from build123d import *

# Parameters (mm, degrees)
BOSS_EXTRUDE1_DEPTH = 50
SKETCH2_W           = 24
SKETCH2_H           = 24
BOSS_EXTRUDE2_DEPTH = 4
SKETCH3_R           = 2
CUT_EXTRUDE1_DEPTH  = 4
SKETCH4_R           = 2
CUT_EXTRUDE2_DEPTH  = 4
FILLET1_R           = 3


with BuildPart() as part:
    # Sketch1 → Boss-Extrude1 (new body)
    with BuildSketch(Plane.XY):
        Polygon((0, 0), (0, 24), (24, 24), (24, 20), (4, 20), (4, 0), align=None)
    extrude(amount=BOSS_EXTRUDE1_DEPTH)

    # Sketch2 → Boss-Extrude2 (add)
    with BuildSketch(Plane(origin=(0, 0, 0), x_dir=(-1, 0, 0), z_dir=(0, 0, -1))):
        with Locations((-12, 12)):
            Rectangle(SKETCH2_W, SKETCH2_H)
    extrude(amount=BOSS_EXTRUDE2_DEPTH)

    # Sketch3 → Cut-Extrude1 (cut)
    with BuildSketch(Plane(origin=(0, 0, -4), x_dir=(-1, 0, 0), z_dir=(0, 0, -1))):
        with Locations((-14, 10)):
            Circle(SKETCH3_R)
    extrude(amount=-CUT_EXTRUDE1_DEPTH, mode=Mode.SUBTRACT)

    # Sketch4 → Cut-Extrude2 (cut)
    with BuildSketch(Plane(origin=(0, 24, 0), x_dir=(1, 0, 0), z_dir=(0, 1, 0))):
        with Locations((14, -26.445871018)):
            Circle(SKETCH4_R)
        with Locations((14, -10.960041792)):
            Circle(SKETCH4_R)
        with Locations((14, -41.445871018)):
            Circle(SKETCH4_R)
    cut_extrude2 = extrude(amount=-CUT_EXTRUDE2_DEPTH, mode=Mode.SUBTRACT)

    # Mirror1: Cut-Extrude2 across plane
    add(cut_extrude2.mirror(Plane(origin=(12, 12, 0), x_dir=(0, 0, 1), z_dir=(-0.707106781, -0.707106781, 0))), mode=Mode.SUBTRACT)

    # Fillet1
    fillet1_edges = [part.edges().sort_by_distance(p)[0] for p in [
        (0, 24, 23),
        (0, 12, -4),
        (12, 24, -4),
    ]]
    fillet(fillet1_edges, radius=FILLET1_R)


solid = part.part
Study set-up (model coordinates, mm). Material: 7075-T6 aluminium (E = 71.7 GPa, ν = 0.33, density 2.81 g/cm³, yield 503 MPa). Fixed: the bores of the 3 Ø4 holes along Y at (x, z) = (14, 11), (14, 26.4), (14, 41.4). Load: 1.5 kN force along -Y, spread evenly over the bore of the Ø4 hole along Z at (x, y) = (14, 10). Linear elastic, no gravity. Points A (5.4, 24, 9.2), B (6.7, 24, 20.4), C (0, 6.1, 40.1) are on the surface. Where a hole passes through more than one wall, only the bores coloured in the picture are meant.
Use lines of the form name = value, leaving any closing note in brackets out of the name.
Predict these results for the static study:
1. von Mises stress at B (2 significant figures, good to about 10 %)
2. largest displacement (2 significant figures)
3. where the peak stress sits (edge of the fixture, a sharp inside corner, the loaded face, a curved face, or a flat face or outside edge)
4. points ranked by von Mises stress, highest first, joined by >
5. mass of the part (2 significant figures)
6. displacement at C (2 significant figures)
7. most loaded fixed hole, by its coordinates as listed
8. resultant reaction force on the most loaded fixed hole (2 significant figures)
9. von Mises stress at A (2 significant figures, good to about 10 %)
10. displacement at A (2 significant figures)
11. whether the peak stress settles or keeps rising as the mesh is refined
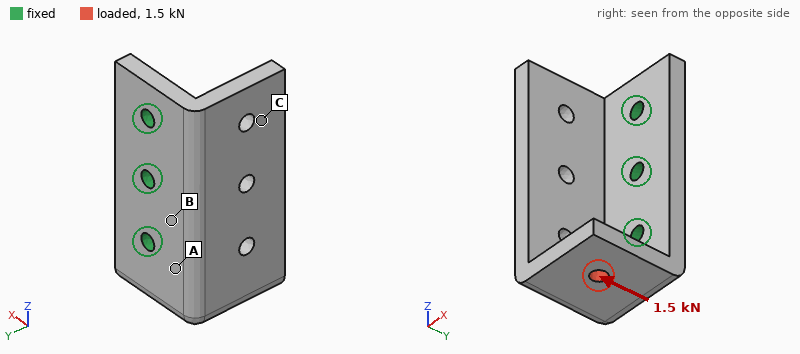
von Mises stress at B = 27 MPa
largest displacement = 0.12 mm
where the peak stress sits = edge of the fixture
points ranked by von Mises stress, highest first, joined by > = A > B > C
mass of the part = 30 g
displacement at C = 0.035 mm
most loaded fixed hole, by its coordinates as listed = (14, 11)
resultant reaction force on the most loaded fixed hole = 1.9 kN
von Mises stress at A = 53 MPa
displacement at A = 0.019 mm
whether the peak stress settles or keeps rising as the mesh is refined = keeps rising
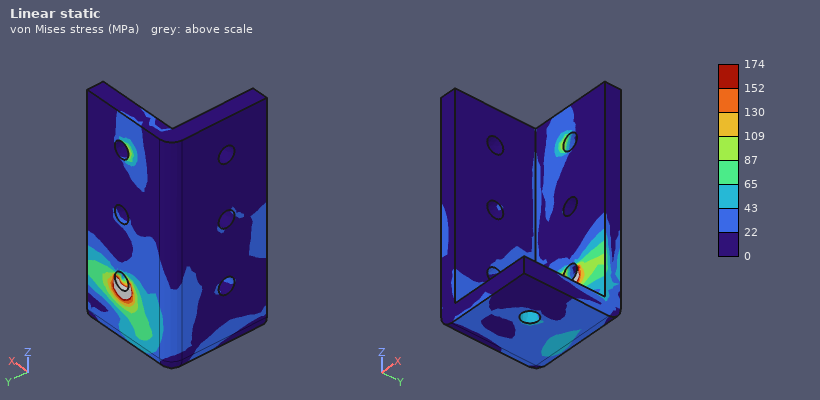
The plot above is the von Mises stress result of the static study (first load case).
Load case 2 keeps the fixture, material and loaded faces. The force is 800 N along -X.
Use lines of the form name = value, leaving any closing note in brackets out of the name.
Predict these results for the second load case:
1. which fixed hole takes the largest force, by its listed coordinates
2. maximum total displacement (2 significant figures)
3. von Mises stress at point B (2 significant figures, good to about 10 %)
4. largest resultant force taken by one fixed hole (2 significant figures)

which fixed hole takes the largest force, by its listed coordinates = (14, 11)
maximum total displacement = 0.14 mm
von Mises stress at point B = 41 MPa
largest resultant force taken by one fixed hole = 1.2 kN
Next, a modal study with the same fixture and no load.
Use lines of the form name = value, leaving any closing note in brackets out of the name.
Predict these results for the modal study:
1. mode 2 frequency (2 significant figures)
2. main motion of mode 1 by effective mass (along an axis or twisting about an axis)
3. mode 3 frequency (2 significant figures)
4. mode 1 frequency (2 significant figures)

mode 2 frequency = 5100 Hz
main motion of mode 1 by effective mass = along X
mode 3 frequency = 7600 Hz
mode 1 frequency = 3900 Hz
